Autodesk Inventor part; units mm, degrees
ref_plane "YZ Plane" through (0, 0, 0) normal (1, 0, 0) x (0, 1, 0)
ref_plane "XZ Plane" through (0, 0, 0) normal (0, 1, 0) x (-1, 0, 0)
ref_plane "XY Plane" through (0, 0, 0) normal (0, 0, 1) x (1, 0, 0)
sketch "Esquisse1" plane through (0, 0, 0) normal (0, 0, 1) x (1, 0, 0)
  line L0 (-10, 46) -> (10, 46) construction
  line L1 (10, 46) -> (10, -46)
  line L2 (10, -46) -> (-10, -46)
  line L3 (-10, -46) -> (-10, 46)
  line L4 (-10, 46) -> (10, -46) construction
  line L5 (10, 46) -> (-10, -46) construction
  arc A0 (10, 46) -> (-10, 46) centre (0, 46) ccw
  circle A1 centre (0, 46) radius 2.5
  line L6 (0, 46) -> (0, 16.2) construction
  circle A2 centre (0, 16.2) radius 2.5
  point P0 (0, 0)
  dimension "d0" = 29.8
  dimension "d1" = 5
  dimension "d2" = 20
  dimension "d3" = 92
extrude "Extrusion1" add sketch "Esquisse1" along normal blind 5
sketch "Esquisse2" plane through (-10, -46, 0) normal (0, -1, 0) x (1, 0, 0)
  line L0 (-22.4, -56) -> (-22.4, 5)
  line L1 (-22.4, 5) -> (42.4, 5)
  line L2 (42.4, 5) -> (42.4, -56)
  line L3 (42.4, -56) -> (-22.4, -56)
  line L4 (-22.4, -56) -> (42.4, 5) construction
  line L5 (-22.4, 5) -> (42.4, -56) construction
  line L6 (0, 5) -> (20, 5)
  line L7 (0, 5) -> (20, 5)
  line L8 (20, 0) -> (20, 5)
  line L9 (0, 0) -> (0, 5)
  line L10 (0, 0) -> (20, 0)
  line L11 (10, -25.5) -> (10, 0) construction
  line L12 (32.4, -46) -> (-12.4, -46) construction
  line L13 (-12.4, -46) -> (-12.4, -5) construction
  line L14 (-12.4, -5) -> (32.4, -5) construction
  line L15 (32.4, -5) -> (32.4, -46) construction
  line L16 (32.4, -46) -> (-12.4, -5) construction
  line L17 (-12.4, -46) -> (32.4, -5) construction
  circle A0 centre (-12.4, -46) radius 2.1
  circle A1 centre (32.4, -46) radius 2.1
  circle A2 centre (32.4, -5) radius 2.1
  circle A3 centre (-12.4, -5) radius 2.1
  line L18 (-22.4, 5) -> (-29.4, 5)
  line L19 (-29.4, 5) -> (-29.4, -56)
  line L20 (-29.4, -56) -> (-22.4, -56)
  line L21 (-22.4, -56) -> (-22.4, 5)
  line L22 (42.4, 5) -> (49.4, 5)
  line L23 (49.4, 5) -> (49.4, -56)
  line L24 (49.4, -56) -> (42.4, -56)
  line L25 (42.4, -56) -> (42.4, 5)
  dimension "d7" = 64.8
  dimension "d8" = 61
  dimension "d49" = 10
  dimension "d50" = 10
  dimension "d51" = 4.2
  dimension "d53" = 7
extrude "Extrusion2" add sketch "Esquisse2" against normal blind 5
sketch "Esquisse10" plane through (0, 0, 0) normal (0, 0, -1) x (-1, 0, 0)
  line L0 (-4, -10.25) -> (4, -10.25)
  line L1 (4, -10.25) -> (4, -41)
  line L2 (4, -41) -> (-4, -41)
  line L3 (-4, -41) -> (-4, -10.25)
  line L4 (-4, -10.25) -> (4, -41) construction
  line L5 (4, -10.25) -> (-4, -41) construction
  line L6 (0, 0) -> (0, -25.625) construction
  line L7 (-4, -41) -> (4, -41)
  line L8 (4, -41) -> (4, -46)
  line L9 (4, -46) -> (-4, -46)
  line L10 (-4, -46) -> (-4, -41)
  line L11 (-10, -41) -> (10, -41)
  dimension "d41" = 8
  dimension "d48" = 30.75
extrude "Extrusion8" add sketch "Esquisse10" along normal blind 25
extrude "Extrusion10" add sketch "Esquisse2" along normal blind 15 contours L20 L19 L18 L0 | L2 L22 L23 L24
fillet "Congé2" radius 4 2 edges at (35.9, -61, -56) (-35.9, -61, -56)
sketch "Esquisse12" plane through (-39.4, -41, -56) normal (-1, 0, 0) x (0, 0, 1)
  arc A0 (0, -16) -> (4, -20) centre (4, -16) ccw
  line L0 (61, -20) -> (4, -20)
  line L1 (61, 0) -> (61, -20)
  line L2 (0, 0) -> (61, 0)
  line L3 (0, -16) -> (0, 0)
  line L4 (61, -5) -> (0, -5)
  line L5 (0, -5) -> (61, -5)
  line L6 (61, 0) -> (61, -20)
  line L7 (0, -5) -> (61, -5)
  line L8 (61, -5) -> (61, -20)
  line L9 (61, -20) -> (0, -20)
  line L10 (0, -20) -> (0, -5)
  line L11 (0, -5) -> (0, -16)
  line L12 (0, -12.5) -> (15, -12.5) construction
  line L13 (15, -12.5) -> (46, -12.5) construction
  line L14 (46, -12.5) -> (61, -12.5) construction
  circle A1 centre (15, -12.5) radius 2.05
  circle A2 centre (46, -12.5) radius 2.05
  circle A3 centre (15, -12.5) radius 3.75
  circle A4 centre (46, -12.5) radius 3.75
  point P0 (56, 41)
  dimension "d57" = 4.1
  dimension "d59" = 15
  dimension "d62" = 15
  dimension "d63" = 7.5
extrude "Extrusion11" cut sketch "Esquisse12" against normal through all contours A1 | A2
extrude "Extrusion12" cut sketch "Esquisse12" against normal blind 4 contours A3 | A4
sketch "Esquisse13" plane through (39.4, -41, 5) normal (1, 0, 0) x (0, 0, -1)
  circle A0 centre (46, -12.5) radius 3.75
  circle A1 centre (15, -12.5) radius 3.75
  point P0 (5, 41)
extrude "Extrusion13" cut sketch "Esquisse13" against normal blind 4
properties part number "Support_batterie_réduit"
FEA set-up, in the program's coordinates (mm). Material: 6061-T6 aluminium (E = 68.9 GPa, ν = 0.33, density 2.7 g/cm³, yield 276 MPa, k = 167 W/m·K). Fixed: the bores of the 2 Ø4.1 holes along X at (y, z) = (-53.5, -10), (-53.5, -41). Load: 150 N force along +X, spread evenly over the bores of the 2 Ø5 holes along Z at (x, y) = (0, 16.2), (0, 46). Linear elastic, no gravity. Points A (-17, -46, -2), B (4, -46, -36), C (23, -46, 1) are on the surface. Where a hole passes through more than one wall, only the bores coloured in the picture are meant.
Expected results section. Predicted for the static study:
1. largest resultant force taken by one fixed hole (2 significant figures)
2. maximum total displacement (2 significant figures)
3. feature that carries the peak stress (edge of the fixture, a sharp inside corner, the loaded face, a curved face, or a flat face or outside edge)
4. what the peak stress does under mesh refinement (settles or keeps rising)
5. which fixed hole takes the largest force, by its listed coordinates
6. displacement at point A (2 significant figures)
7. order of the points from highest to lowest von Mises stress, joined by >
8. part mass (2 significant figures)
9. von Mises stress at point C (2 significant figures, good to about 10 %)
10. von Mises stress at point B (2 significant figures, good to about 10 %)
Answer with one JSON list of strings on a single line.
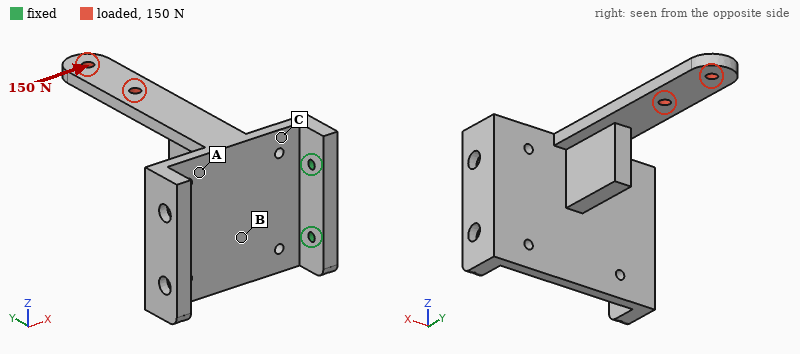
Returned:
["210 N", "1.5 mm", "edge of the fixture", "keeps rising", "(-53.5, -10)", "0.51 mm", "C > B > A", "140 g", "54 MPa", "30 MPa"]
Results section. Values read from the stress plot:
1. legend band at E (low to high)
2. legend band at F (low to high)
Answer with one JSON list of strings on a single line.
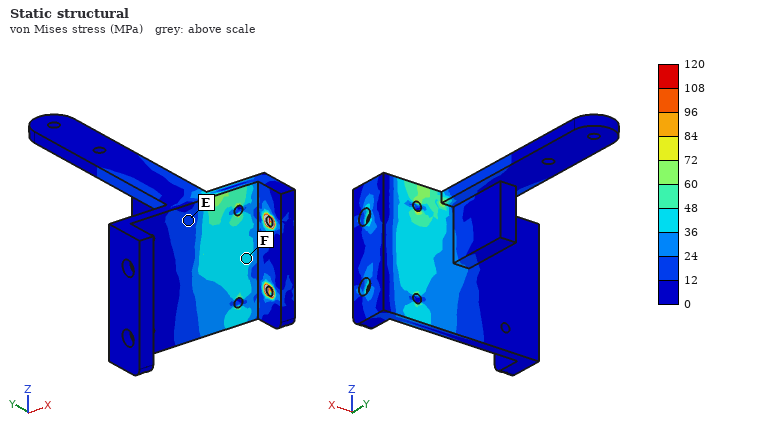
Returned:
["12 to 24 MPa", "36 to 48 MPa"]
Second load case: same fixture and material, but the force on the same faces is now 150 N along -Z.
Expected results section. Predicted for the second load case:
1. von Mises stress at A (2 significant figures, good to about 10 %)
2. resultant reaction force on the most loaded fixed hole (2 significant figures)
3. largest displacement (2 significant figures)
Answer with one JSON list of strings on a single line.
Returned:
["6.7 MPa", "430 N", "0.98 mm"]
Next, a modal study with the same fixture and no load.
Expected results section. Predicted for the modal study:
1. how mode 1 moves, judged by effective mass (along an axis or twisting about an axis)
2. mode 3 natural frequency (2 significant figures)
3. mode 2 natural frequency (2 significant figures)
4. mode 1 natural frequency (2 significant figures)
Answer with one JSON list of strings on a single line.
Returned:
["along Y", "1200 Hz", "650 Hz", "310 Hz"]
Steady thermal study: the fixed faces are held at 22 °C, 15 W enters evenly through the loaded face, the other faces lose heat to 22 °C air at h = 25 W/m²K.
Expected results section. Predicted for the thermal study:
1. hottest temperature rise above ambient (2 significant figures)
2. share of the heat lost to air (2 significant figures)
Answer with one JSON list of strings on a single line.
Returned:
["53 K", "43 %"]
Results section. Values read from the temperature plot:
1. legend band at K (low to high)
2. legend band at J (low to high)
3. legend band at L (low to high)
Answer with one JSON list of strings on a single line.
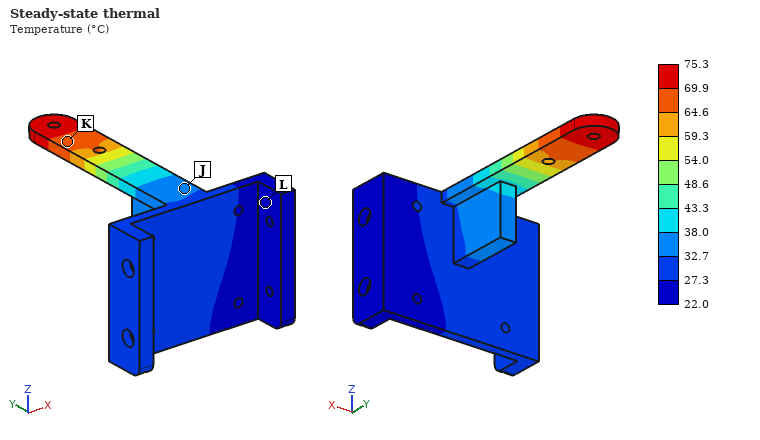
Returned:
["64.6 to 69.9 °C", "32.7 to 38.0 °C", "22.0 to 27.3 °C"]
